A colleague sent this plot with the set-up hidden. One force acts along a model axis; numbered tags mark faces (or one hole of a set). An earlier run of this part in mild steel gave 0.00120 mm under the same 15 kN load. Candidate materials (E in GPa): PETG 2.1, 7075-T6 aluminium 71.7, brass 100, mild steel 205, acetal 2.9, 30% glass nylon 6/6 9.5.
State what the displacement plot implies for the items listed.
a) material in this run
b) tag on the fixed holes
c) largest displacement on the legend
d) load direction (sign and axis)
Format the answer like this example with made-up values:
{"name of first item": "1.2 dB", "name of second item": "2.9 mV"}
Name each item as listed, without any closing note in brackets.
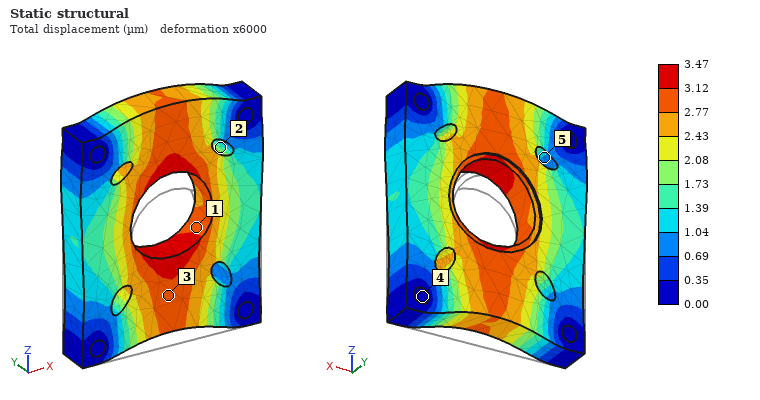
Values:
{"material in this run": "7075-T6 aluminium", "tag on the fixed holes": "4", "largest displacement on the legend": "3.47 µm", "load direction": "+Z"}
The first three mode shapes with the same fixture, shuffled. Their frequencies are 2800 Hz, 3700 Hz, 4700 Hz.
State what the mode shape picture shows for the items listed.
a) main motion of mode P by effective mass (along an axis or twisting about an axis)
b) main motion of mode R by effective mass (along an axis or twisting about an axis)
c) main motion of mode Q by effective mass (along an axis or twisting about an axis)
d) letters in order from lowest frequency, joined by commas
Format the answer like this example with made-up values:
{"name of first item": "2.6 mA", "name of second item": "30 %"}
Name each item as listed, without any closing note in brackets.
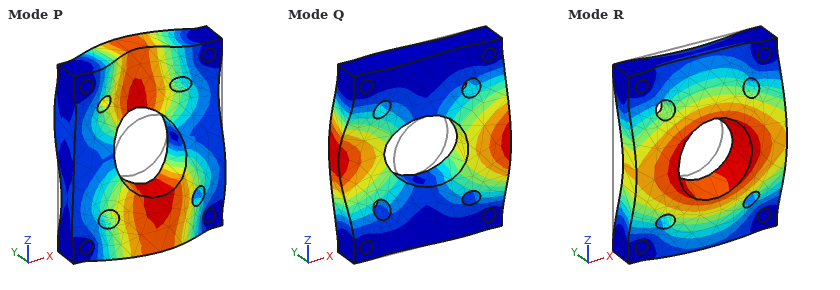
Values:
{"main motion of mode P by effective mass": "twisting about X", "main motion of mode R by effective mass": "along Y", "main motion of mode Q by effective mass": "twisting about Z", "letters in order from lowest frequency, joined by commas": "R, Q, P"}
